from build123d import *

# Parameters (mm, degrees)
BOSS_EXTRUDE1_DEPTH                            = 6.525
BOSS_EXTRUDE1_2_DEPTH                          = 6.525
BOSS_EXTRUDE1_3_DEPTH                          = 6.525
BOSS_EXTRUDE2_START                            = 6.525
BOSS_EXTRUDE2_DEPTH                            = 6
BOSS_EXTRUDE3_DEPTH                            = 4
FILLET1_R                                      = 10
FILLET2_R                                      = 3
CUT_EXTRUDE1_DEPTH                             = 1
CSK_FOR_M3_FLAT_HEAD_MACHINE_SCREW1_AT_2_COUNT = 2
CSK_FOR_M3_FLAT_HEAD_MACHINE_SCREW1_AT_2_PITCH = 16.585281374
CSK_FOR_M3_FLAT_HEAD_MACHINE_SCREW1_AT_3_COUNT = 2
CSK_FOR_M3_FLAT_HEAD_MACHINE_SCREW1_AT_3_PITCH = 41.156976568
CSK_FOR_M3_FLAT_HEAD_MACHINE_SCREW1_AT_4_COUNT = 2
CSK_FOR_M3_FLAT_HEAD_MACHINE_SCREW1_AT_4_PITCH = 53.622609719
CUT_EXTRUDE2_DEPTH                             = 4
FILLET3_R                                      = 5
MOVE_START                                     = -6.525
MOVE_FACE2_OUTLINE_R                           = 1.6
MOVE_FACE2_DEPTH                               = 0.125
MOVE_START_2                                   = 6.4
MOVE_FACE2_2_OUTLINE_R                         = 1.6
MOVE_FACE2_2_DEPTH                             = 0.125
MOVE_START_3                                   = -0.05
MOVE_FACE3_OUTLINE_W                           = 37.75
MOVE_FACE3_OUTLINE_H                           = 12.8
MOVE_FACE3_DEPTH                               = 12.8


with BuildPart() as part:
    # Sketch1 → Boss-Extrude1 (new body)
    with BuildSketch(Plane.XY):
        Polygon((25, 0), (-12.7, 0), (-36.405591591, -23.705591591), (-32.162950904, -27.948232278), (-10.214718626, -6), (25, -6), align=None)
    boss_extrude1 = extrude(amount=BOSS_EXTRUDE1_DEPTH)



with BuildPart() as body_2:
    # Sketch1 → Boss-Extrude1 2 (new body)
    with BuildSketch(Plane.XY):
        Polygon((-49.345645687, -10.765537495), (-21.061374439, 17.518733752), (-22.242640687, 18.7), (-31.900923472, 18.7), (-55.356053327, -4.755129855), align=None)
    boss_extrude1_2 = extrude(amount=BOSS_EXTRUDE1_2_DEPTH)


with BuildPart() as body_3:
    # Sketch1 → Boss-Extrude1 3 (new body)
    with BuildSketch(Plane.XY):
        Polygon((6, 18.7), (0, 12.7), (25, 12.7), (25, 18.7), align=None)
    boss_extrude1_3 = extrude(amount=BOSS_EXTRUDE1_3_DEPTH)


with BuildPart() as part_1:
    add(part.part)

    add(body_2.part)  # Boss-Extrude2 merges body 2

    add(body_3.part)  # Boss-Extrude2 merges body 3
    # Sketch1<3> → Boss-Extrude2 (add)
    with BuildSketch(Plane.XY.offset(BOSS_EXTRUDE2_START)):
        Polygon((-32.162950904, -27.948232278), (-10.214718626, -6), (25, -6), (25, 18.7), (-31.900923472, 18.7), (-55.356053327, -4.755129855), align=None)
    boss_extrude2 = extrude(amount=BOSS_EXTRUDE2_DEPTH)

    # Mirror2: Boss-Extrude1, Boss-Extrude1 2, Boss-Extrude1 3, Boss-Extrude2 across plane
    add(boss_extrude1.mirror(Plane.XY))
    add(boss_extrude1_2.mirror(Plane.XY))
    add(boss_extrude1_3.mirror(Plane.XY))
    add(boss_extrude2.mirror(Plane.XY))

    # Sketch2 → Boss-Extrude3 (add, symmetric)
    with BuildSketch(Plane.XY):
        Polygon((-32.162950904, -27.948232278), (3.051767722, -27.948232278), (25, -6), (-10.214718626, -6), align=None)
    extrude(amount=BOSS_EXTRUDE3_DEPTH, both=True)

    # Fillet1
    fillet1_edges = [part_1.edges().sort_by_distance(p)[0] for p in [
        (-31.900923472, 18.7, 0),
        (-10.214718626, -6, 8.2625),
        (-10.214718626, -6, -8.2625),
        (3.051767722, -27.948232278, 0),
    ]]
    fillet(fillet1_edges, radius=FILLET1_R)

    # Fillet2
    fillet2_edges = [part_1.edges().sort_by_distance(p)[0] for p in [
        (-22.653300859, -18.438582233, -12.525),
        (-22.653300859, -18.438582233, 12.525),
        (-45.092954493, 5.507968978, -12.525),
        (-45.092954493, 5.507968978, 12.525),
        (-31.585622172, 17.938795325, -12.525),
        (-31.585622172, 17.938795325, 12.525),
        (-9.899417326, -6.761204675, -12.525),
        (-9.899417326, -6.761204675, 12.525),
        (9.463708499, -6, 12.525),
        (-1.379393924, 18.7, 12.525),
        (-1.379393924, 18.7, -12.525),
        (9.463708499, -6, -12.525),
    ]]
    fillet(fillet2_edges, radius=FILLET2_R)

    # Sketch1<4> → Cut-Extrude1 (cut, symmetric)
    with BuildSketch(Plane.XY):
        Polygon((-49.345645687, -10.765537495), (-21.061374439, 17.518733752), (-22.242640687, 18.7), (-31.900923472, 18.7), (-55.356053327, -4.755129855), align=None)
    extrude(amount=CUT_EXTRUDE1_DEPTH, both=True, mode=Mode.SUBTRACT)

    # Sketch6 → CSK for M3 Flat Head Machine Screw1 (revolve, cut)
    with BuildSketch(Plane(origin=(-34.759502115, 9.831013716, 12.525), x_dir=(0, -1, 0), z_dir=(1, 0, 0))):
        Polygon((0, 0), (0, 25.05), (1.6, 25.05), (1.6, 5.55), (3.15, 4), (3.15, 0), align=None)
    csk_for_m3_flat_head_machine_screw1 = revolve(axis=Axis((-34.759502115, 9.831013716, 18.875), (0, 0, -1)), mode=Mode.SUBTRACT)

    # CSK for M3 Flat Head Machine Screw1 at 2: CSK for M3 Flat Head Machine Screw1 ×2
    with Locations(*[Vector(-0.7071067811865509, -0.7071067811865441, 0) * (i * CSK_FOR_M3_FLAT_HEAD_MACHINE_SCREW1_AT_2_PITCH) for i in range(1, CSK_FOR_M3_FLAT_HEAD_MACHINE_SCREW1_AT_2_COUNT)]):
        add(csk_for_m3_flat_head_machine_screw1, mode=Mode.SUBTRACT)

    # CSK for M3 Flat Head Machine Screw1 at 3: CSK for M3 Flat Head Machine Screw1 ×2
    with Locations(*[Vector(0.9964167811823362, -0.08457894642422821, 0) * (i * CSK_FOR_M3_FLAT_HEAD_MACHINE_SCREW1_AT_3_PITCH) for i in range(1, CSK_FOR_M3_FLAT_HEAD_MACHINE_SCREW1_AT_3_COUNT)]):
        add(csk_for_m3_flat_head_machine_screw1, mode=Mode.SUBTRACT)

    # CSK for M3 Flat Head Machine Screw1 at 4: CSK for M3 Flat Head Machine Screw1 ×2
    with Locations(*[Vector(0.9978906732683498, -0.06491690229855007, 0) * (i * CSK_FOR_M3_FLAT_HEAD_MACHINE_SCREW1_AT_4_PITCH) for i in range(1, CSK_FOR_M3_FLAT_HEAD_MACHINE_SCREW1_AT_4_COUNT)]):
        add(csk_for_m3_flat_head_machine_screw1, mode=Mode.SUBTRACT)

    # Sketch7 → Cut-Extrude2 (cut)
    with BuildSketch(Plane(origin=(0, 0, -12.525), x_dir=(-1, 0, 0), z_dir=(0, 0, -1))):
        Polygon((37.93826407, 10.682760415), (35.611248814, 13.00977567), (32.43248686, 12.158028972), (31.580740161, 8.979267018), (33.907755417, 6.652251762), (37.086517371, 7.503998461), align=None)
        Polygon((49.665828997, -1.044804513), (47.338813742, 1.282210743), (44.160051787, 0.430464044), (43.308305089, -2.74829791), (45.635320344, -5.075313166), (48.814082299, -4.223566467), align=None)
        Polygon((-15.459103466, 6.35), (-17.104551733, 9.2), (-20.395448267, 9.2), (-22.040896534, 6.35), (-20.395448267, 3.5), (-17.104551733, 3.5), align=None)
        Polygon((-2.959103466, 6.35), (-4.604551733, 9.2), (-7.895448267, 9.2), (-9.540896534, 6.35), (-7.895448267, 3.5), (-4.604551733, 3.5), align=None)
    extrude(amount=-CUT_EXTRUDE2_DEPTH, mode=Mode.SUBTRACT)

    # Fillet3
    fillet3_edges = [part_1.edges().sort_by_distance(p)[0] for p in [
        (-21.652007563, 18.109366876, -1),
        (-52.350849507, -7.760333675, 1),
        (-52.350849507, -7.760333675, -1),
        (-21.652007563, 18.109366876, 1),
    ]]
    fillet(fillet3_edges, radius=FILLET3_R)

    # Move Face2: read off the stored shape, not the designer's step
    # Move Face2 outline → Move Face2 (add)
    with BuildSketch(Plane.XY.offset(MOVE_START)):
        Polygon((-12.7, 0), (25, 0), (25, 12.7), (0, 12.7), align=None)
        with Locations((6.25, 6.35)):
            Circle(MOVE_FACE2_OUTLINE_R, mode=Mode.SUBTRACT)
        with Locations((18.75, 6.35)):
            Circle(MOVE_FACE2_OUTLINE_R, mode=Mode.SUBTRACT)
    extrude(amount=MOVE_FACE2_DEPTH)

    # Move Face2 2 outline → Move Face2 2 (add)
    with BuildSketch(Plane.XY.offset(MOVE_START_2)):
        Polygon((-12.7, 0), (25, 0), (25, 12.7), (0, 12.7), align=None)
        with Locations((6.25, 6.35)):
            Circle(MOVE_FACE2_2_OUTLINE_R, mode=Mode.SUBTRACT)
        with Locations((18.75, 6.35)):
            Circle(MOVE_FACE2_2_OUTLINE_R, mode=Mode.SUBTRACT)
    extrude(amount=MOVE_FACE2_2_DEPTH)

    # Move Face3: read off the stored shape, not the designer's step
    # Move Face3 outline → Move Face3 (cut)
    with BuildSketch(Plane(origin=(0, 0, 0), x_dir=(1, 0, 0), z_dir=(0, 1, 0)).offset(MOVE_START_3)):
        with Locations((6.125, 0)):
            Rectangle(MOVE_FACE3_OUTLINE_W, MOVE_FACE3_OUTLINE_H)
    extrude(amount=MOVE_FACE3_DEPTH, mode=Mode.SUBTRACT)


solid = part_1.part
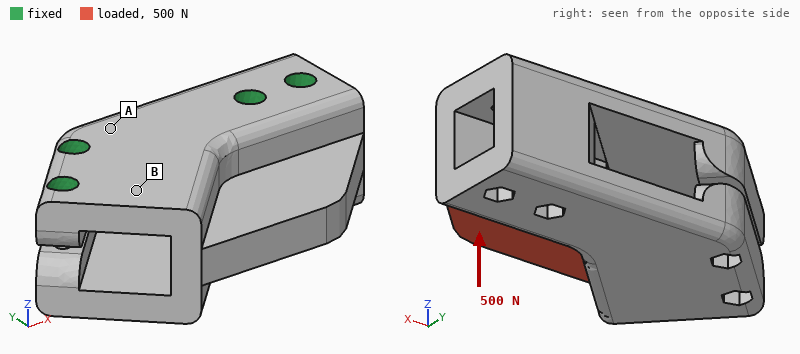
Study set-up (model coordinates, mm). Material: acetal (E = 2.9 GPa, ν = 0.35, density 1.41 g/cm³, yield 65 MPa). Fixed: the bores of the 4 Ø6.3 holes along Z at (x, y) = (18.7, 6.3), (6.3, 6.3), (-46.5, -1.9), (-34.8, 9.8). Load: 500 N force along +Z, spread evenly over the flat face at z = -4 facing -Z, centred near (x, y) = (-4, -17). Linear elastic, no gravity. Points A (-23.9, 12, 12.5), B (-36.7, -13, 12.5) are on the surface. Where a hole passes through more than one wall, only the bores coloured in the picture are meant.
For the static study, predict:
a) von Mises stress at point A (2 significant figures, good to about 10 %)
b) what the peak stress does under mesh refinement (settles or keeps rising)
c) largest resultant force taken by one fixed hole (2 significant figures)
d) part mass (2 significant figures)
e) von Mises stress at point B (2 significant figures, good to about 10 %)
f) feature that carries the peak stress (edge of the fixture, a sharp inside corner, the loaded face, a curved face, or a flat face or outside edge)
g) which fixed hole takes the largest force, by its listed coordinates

3.5 MPa
keeps rising
290 N
58 g
7.8 MPa
edge of the fixture
(6.3, 6.3)
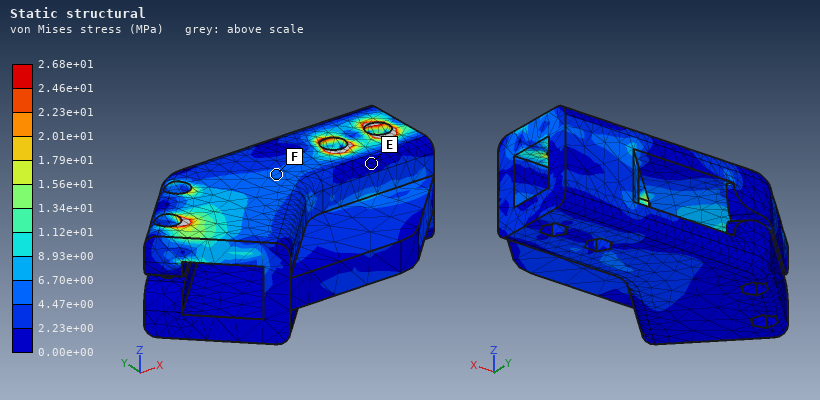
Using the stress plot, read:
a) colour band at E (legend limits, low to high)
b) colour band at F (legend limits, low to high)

0.00e+00 to 2.23e+00 MPa
4.47e+00 to 6.70e+00 MPa
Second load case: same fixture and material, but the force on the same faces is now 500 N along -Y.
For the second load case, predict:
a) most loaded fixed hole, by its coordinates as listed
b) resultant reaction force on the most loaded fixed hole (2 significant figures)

(6.3, 6.3)
320 N
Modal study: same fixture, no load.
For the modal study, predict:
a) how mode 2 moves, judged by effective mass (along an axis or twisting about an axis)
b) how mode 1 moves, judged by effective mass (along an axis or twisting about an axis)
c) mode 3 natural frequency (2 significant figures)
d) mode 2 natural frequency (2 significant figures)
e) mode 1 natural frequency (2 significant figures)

along Z
along Y
1900 Hz
940 Hz
860 Hz
